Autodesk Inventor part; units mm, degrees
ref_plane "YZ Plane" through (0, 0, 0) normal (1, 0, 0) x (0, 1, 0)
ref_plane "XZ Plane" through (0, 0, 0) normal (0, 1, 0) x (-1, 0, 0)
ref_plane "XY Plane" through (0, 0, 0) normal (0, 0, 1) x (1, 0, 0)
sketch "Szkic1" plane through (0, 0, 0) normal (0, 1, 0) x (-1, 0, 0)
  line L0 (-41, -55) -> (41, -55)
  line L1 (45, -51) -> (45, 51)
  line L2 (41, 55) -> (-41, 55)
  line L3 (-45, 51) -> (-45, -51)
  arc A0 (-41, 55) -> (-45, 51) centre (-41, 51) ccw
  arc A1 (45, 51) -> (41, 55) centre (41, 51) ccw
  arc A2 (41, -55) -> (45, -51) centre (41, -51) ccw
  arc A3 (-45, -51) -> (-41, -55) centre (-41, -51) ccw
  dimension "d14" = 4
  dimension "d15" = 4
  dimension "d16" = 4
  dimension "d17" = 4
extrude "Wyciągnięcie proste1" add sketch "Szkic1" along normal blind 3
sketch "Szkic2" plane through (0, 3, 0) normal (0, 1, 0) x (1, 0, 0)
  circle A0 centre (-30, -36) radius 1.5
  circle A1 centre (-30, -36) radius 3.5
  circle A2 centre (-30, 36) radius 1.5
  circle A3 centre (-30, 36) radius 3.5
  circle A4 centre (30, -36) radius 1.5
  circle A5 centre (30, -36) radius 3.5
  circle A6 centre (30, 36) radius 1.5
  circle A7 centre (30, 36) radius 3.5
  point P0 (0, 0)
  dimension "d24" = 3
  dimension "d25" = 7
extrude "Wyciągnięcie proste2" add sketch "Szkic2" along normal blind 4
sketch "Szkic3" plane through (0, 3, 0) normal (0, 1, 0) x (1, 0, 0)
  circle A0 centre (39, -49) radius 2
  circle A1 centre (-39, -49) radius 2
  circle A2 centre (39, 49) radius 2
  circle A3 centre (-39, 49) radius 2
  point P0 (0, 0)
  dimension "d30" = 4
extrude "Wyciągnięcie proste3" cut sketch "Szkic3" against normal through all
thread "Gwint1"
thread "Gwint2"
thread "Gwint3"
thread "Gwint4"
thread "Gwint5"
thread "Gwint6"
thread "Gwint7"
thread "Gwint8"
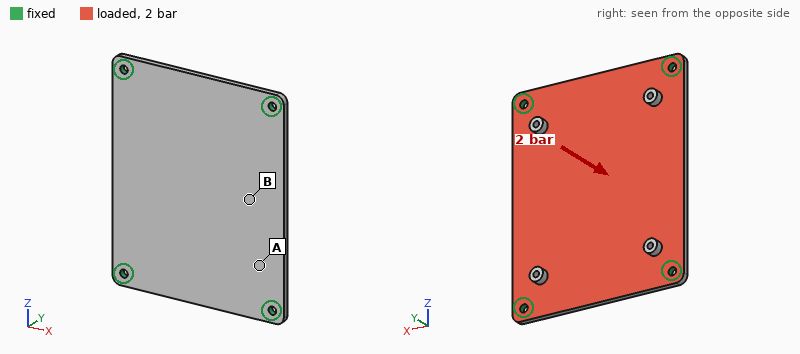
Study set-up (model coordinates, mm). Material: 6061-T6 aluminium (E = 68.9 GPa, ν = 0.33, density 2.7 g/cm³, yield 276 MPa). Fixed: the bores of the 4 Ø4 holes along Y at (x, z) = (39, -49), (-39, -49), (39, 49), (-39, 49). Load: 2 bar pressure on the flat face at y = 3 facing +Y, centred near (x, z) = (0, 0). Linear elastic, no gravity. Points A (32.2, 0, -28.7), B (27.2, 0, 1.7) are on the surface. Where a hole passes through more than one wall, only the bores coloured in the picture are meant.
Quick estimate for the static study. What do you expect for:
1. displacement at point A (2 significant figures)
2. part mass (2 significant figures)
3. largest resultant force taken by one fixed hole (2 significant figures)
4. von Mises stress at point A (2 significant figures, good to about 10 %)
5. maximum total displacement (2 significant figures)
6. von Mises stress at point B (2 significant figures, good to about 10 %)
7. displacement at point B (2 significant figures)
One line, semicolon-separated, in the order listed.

0.25 mm; 81 g; 480 N; 20 MPa; 0.59 mm; 64 MPa; 0.51 mm
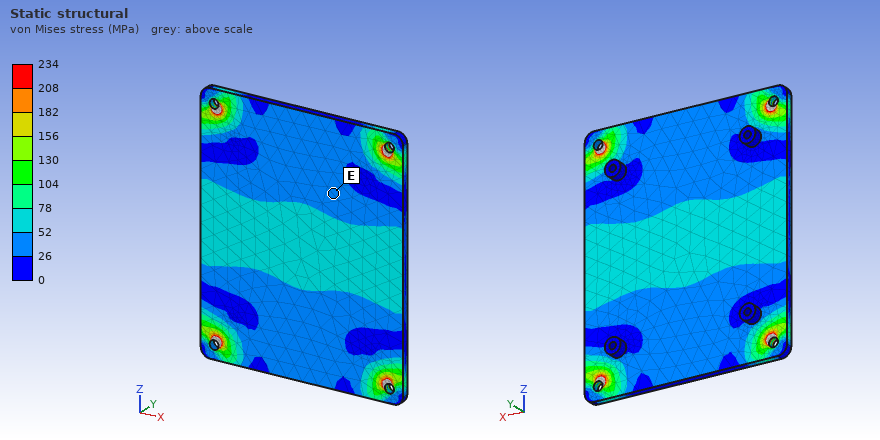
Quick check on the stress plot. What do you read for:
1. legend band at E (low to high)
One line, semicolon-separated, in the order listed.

26 to 52 MPa
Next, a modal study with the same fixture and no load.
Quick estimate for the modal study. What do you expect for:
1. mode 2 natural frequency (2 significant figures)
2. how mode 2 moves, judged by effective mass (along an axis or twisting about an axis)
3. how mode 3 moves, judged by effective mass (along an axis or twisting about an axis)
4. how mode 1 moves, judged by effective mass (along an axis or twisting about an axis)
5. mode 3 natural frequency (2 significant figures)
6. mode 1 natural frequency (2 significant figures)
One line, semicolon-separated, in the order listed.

2000 Hz; twisting about Z; twisting about X; along Y; 2500 Hz; 1200 Hz
